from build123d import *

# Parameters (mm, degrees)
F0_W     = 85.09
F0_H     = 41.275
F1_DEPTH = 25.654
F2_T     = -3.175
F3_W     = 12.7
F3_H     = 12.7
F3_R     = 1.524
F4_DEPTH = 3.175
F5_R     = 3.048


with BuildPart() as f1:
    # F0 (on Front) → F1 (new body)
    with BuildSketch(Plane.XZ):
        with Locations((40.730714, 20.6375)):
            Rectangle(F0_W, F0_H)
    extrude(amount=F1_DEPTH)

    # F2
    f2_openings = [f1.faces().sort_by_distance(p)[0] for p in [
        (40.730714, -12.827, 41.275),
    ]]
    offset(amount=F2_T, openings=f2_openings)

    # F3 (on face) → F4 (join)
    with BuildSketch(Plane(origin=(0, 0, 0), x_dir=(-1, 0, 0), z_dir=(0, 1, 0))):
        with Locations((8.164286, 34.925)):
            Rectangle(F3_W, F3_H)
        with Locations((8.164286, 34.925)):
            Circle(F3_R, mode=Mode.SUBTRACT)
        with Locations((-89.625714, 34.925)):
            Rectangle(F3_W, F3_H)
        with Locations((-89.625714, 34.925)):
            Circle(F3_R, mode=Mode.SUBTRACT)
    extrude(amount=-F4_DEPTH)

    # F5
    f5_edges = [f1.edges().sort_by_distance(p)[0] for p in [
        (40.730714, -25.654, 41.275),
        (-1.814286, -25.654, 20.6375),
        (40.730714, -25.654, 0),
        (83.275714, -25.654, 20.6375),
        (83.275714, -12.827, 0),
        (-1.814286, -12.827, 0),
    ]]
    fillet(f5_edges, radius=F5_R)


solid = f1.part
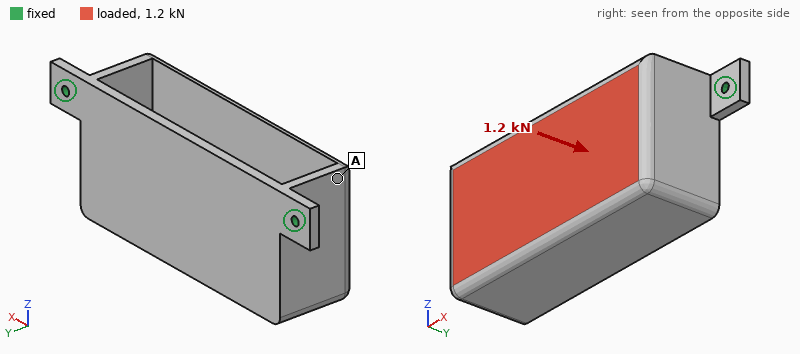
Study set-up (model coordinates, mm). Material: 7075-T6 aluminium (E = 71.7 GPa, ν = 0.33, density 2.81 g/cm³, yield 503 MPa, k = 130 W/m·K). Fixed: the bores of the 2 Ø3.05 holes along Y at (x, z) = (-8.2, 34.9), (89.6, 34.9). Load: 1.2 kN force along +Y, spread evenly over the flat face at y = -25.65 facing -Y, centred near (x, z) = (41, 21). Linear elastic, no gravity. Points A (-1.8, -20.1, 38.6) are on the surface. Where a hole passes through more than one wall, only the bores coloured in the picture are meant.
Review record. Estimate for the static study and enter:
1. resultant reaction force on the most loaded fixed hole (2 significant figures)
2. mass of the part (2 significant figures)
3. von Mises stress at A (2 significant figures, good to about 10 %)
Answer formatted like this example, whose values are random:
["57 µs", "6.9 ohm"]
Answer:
["610 N", "92 g", "46 MPa"]
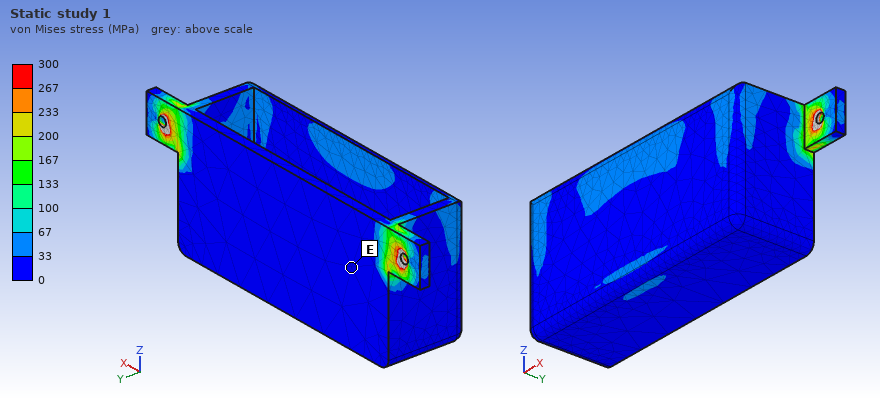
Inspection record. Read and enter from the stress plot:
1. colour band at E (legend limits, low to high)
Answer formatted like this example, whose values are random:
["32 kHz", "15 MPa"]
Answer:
["0 to 33 MPa"]
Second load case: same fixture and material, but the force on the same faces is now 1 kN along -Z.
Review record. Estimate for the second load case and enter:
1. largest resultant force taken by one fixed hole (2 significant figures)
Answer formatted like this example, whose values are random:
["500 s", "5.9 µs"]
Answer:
["500 N"]
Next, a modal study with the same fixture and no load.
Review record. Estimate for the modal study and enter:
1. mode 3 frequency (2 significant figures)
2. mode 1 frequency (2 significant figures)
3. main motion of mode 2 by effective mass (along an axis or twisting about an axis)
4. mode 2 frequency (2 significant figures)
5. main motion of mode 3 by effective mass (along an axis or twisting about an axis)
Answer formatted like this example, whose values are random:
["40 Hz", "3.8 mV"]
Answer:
["2700 Hz", "690 Hz", "along X", "1800 Hz", "along Y"]
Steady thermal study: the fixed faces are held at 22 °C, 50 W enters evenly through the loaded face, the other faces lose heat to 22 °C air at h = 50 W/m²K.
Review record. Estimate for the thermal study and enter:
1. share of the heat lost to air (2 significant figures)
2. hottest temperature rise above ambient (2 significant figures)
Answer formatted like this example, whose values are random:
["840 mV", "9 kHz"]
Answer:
["57 %", "52 K"]
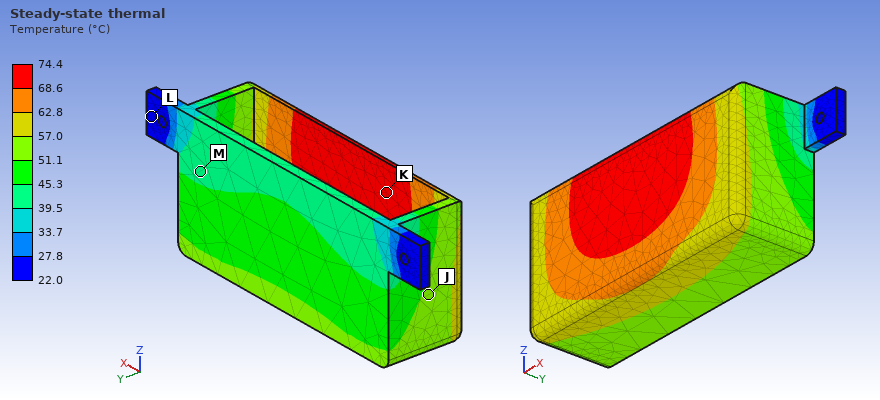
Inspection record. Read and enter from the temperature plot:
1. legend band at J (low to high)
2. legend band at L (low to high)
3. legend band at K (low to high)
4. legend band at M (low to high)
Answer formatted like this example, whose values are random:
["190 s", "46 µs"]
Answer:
["51.1 to 57.0 °C", "22.0 to 27.8 °C", "68.6 to 74.4 °C", "39.5 to 45.3 °C"]
